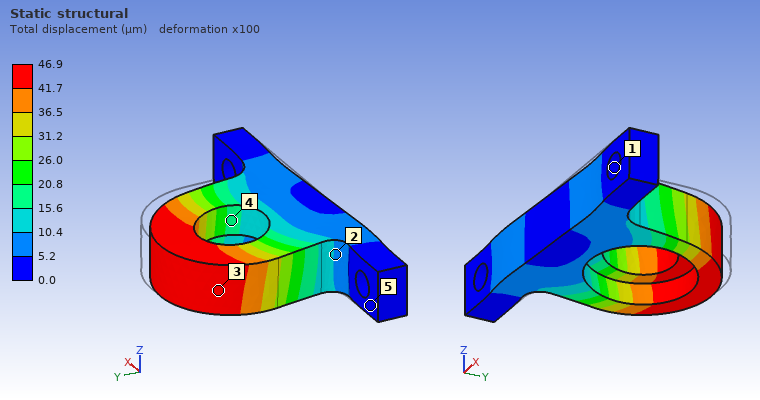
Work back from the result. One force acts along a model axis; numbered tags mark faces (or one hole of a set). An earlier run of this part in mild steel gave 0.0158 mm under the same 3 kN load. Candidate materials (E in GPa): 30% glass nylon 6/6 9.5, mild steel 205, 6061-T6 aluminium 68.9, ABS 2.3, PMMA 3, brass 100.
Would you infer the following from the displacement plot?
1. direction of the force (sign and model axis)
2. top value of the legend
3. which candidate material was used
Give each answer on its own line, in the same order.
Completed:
-X
46.9 µm
6061-T6 aluminium
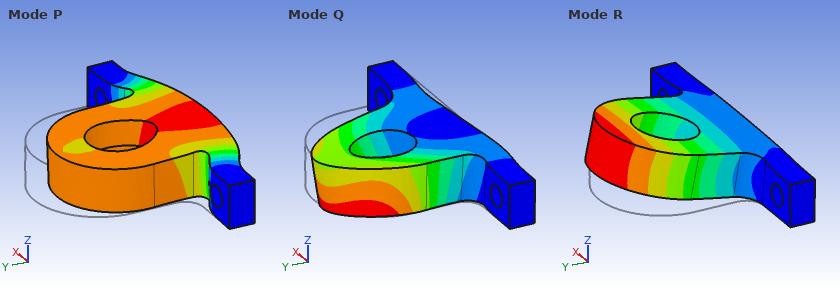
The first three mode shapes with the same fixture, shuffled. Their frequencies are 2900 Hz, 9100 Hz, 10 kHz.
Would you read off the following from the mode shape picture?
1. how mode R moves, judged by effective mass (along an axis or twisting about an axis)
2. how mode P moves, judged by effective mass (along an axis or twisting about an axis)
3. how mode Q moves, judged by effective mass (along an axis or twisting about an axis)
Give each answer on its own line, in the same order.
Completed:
along Z
along Y
along X
